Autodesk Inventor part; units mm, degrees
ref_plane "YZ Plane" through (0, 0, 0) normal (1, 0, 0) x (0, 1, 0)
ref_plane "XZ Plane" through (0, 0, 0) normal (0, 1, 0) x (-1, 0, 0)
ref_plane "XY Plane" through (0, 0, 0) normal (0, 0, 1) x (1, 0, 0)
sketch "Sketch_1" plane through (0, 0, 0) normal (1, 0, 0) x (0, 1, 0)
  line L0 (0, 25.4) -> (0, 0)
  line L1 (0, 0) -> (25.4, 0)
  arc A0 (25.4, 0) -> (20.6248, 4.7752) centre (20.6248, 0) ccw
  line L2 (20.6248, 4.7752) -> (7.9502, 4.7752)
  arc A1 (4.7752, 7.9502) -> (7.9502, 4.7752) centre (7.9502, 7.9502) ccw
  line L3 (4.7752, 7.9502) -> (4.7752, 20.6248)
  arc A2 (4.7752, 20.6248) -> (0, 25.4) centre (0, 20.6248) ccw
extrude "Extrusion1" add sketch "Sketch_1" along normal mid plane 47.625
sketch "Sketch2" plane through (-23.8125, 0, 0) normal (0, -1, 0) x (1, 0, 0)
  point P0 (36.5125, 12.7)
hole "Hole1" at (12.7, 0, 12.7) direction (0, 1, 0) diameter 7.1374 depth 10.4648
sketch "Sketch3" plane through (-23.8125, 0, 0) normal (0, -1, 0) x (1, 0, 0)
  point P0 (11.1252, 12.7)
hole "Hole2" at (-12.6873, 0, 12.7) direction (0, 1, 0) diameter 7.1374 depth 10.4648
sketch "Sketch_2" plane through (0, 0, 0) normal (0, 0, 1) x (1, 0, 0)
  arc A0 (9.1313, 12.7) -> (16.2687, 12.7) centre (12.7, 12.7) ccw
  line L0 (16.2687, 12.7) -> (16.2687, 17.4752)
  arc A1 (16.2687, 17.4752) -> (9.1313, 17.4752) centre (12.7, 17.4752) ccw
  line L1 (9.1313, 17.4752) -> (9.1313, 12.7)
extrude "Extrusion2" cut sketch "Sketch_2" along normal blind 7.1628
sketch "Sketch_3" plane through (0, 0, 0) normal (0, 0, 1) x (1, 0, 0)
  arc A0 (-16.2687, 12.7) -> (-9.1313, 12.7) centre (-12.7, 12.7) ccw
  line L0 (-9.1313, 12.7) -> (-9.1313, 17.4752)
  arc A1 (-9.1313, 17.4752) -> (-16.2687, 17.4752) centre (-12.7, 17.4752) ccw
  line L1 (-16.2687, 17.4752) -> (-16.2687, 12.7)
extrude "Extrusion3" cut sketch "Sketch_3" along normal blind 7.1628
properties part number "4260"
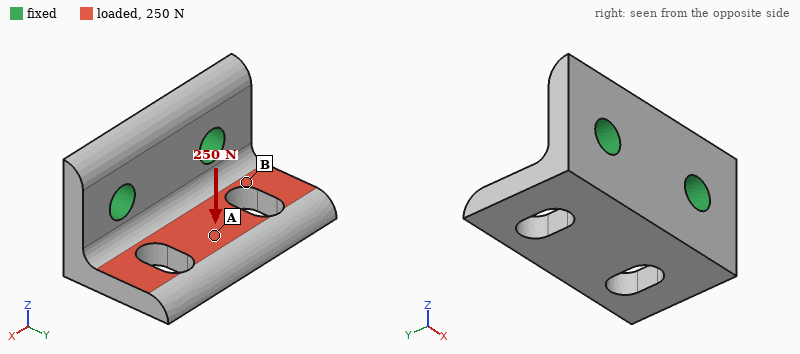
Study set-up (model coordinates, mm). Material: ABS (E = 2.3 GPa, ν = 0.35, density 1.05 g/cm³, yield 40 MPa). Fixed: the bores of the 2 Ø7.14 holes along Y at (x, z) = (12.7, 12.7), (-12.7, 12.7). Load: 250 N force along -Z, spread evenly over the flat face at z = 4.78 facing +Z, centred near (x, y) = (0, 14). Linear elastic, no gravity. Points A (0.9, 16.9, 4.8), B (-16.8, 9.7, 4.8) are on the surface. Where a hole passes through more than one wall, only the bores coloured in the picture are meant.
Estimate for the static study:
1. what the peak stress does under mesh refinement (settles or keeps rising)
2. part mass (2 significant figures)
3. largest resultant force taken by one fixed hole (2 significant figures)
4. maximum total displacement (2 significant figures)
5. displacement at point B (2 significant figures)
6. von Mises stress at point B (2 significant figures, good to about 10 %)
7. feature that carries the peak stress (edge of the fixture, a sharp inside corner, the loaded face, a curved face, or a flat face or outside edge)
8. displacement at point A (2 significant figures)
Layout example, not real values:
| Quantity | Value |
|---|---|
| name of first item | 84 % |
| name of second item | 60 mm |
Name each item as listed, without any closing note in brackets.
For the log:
| Quantity | Value |
|---|---|
| what the peak stress does under mesh refinement | keeps rising |
| part mass | 9.5 g |
| largest resultant force taken by one fixed hole | 130 N |
| maximum total displacement | 0.69 mm |
| displacement at point B | 0.16 mm |
| von Mises stress at point B | 8.6 MPa |
| feature that carries the peak stress | edge of the fixture |
| displacement at point A | 0.39 mm |
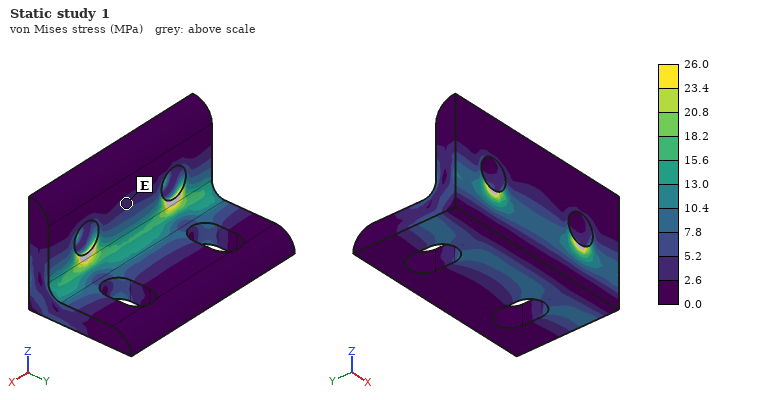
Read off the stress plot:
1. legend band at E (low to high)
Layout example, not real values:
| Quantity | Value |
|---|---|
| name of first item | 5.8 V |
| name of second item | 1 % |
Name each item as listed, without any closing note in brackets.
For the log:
| Quantity | Value |
|---|---|
| legend band at E | 2.6 to 5.2 MPa |
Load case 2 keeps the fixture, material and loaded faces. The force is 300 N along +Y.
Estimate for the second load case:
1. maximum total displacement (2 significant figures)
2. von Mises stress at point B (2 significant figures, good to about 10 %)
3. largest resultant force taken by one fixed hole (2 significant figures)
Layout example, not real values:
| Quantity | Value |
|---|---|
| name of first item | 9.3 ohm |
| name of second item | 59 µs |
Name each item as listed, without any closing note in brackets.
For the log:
| Quantity | Value |
|---|---|
| maximum total displacement | 81 µm |
| von Mises stress at point B | 6.3 MPa |
| largest resultant force taken by one fixed hole | 150 N |
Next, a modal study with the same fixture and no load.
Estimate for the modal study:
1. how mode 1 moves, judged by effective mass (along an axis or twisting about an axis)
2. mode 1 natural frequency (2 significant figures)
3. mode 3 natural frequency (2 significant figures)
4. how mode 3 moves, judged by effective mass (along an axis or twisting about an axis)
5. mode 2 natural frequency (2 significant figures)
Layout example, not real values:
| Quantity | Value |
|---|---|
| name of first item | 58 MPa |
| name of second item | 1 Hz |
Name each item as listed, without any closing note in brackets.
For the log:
| Quantity | Value |
|---|---|
| how mode 1 moves, judged by effective mass | along Z |
| mode 1 natural frequency | 1700 Hz |
| mode 3 natural frequency | 4300 Hz |
| how mode 3 moves, judged by effective mass | along X |
| mode 2 natural frequency | 2600 Hz |
